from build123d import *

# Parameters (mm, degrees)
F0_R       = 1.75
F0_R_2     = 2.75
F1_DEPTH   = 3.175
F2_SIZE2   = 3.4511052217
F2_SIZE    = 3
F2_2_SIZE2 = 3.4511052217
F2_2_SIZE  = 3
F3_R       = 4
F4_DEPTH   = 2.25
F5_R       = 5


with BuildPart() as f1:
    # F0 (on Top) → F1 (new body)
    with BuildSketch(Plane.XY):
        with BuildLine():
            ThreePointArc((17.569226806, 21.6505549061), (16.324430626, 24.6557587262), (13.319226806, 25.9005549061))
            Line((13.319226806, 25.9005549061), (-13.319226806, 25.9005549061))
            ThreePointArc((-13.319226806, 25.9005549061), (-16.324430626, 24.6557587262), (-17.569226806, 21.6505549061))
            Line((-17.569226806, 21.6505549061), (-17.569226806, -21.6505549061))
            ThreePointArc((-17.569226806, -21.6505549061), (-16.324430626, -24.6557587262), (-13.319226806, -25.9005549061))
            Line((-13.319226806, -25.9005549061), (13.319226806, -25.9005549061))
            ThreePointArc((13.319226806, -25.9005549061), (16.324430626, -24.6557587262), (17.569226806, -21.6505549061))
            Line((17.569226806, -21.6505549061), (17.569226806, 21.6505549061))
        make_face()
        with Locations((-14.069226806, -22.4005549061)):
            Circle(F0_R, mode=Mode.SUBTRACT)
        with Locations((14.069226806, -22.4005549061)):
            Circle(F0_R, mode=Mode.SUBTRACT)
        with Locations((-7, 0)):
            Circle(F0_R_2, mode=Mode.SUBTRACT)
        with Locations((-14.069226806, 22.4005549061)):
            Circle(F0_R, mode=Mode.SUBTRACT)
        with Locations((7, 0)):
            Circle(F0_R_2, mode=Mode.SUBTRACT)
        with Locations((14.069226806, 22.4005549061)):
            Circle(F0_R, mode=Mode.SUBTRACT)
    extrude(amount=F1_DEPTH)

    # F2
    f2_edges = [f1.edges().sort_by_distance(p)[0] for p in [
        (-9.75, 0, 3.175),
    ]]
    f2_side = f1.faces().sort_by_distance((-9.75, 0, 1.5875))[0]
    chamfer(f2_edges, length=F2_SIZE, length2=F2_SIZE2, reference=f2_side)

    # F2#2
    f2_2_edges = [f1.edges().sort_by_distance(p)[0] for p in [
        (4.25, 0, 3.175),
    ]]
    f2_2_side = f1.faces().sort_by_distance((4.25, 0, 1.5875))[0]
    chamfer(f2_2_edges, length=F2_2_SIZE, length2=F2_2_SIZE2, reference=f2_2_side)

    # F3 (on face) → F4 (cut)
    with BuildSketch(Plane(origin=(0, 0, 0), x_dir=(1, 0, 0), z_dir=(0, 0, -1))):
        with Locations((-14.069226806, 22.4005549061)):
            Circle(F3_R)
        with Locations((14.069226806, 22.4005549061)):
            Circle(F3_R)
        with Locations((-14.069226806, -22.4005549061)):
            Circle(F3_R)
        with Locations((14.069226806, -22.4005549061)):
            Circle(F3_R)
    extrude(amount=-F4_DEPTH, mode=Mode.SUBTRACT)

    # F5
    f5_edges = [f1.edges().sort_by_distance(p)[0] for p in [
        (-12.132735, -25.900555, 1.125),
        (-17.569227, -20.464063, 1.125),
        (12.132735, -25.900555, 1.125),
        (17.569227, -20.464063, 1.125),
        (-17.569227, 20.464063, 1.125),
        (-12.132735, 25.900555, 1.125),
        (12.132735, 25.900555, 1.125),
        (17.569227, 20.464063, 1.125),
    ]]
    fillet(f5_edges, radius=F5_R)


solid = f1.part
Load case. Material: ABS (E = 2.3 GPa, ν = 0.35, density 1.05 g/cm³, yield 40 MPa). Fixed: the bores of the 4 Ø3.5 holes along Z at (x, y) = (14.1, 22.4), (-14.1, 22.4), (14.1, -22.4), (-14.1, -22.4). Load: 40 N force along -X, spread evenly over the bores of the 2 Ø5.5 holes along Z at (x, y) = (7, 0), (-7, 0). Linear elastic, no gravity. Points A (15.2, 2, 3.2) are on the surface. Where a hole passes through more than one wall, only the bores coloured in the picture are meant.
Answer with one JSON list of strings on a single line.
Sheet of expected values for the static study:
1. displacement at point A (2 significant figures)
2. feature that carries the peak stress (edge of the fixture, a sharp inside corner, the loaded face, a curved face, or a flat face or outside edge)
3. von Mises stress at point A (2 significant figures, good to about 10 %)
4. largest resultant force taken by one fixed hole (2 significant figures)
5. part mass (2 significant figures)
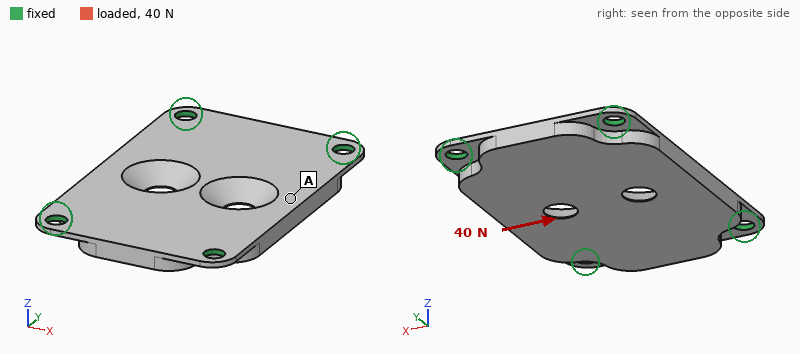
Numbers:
["14 µm", "the loaded face", "0.66 MPa", "12 N", "5.0 g"]
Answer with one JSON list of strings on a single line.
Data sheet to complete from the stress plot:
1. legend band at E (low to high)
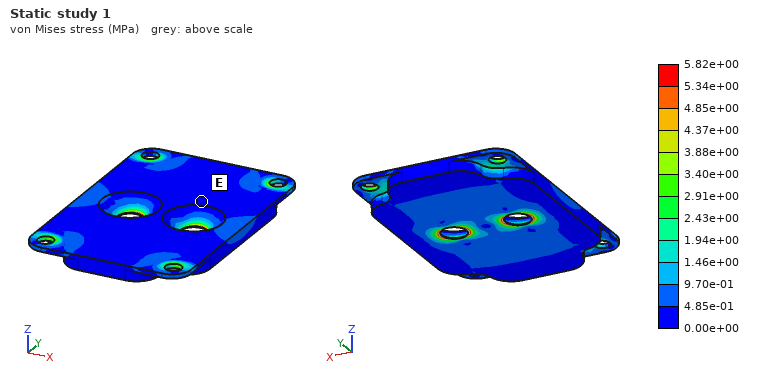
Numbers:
["0.00e+00 to 4.85e-01 MPa"]
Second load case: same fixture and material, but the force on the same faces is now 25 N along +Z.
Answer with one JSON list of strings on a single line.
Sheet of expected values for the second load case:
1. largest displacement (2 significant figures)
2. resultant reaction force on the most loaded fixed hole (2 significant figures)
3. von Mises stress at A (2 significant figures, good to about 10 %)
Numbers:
["0.18 mm", "27 N", "3.7 MPa"]
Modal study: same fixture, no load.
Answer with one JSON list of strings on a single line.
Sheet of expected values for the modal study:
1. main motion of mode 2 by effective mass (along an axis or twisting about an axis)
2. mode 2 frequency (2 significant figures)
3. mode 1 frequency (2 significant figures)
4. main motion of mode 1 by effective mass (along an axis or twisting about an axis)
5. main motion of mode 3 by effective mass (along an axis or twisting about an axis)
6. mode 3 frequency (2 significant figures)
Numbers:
["twisting about Y", "2400 Hz", "1500 Hz", "along Z", "twisting about X", "3500 Hz"]
